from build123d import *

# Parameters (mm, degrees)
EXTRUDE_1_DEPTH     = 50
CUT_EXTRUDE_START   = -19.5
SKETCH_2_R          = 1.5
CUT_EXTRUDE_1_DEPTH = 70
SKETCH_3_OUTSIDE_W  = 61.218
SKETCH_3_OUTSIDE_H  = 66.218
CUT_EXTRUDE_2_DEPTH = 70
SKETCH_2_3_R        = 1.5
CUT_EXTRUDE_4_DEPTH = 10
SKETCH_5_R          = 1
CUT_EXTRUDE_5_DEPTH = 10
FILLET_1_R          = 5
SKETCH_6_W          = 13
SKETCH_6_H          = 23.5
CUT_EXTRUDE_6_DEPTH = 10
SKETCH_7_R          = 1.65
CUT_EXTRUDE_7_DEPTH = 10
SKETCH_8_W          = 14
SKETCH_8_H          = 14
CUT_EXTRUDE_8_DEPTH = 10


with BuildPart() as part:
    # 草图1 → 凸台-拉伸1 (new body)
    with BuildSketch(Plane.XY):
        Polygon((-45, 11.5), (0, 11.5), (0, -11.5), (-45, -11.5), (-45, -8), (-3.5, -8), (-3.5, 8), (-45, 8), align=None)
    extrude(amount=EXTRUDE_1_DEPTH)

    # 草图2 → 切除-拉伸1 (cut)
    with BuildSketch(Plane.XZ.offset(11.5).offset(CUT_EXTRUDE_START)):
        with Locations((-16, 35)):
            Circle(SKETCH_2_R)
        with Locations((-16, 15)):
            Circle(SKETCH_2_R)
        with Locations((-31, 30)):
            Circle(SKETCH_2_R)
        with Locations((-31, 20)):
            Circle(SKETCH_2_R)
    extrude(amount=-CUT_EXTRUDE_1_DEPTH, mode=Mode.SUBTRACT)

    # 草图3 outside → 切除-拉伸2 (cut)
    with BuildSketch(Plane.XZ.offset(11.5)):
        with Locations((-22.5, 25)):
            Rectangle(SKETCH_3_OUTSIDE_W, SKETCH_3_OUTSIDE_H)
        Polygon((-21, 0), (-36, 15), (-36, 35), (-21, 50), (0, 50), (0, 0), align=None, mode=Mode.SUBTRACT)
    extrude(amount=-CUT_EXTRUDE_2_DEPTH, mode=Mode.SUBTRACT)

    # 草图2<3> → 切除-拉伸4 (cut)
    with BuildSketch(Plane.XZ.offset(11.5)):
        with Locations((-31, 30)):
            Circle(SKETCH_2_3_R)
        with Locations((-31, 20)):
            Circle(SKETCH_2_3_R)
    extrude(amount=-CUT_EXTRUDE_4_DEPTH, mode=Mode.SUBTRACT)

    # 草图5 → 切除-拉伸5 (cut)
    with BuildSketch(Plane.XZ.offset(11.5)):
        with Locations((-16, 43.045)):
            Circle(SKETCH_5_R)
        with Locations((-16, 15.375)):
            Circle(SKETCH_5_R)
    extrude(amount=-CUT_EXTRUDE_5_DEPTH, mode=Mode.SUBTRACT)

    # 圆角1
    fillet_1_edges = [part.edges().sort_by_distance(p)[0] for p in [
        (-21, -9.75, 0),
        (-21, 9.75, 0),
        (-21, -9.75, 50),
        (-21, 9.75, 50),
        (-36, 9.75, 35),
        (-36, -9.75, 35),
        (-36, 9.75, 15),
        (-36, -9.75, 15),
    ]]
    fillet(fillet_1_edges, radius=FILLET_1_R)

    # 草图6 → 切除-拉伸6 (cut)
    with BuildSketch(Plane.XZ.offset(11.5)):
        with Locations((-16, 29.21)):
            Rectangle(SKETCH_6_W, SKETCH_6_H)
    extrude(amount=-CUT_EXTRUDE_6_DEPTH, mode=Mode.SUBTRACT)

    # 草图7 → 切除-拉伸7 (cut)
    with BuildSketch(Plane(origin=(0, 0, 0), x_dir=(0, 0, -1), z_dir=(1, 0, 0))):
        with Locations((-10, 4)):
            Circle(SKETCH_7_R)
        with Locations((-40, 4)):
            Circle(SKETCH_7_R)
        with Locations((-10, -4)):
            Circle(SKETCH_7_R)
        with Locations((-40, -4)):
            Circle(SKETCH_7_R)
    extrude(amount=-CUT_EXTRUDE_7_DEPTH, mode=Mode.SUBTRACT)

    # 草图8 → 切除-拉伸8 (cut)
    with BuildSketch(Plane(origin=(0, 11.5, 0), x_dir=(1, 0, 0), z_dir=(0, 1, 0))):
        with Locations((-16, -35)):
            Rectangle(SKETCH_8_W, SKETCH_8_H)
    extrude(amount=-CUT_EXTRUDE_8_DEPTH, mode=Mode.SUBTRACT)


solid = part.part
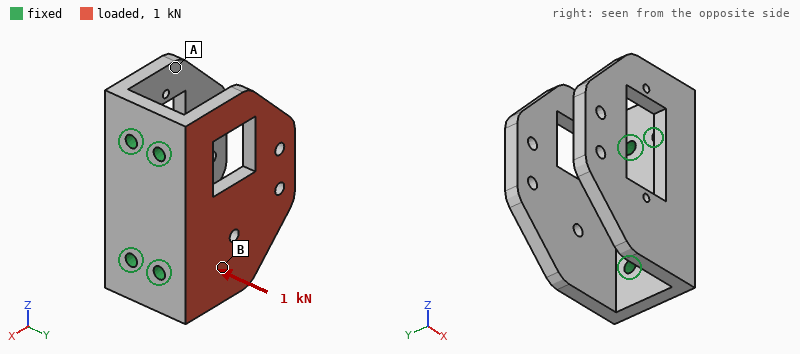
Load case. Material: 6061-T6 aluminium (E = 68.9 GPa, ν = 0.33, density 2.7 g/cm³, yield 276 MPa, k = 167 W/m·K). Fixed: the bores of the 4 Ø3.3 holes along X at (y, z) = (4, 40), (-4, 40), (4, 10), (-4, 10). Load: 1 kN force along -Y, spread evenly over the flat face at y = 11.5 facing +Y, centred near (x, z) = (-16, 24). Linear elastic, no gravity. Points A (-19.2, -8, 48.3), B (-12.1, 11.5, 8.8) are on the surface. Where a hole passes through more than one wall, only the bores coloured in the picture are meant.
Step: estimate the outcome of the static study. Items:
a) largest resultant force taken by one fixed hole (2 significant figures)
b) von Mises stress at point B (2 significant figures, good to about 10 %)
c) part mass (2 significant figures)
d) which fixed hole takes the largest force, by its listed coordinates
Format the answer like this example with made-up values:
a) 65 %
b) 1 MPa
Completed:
a) 570 N
b) 76 MPa
c) 32 g
d) (4, 10)
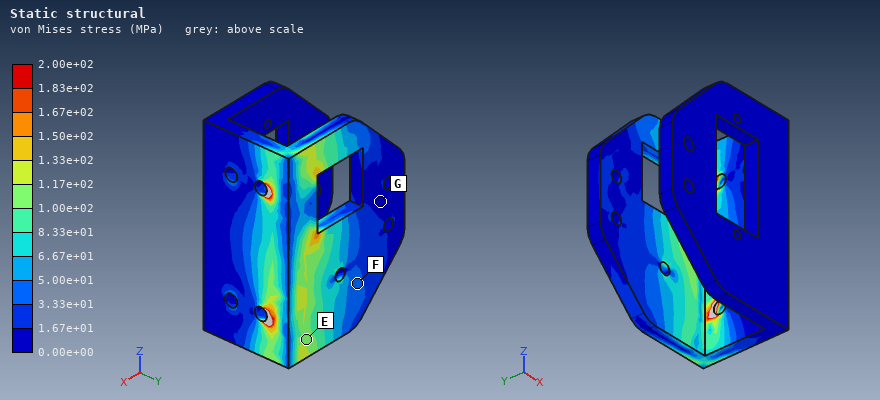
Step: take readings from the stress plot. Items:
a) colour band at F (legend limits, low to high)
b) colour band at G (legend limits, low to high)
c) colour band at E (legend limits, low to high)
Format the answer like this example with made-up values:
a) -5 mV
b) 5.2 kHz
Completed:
a) 3.33e+01 to 5.00e+01 MPa
b) 0.00e+00 to 1.67e+01 MPa
c) 1.00e+02 to 1.17e+02 MPa
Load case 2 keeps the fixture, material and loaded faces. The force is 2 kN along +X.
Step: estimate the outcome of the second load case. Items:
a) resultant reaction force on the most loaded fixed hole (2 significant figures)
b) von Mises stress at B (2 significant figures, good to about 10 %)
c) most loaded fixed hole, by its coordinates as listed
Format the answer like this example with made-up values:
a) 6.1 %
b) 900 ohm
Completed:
a) 1.4 kN
b) 37 MPa
c) (4, 10)
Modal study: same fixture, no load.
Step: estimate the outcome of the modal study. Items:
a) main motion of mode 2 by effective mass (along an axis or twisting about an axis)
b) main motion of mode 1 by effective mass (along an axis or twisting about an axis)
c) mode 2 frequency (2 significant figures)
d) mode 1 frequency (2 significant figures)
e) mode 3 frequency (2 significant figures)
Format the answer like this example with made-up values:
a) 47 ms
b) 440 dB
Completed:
a) along Y
b) along Y
c) 2300 Hz
d) 2100 Hz
e) 5000 Hz
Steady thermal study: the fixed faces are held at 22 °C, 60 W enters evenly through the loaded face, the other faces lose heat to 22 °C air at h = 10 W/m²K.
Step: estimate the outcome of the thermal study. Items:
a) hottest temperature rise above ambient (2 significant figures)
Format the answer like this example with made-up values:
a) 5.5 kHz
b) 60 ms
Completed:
a) 58 K
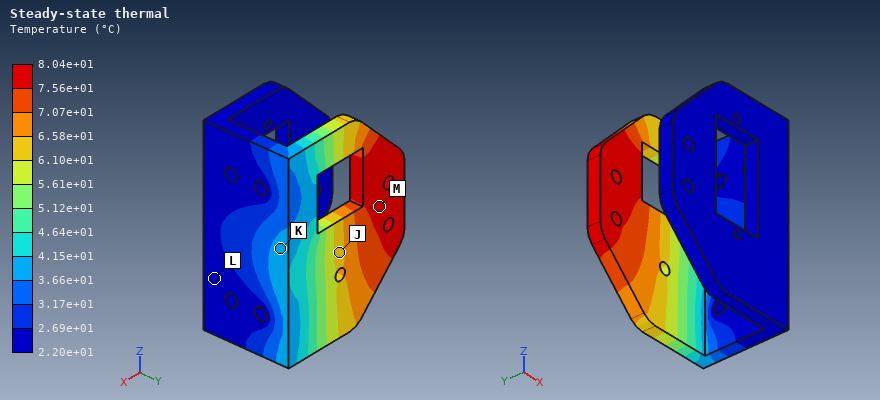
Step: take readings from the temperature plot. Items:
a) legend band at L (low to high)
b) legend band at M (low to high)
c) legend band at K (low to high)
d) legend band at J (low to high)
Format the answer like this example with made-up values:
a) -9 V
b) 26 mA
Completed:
a) 2.20e+01 to 2.69e+01 °C
b) 7.56e+01 to 8.04e+01 °C
c) 3.66e+01 to 4.15e+01 °C
d) 6.10e+01 to 6.58e+01 °C
